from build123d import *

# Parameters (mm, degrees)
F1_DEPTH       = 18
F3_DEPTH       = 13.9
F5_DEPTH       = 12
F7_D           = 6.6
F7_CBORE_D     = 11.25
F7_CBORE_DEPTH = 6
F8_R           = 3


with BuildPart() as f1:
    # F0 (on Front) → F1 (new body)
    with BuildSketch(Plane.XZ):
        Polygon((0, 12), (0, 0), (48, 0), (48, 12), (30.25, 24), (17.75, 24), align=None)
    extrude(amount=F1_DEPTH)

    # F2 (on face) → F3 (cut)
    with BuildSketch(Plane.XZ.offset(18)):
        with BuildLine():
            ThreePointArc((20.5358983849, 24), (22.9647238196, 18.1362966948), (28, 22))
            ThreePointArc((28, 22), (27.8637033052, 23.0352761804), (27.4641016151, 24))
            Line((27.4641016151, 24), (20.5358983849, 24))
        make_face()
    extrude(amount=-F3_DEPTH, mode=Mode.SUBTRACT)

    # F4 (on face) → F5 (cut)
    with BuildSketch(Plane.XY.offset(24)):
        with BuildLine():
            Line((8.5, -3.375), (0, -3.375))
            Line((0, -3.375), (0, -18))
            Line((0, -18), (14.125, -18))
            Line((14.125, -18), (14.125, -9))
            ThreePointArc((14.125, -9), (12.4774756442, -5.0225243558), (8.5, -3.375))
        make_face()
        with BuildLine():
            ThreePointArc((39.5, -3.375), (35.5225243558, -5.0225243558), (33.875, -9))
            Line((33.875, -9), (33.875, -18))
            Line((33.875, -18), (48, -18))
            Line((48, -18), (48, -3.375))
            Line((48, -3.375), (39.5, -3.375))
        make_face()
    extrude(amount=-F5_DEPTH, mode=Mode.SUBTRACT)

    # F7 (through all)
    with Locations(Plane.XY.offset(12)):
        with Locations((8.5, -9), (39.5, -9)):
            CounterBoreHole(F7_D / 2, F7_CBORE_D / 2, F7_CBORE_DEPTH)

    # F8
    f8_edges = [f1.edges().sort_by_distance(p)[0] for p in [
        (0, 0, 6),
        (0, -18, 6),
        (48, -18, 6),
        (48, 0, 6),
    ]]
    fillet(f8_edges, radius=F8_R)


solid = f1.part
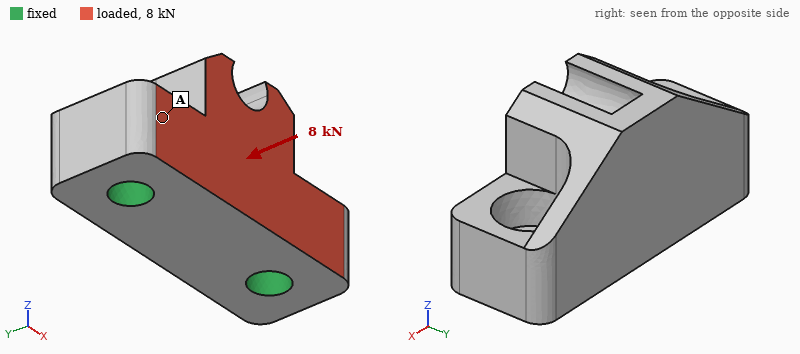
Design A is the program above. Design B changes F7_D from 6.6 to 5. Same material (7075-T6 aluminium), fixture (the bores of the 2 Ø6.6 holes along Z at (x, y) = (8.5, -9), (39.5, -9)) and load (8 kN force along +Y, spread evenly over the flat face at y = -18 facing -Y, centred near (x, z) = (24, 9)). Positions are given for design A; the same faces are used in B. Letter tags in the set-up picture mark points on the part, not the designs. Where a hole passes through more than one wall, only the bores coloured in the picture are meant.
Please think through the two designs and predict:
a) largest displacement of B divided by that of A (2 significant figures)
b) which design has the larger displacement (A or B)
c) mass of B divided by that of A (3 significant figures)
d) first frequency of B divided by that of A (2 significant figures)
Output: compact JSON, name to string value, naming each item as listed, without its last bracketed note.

{"largest displacement of B divided by that of A": "1.3", "which design has the larger displacement": "B", "mass of B divided by that of A": "1.01", "first frequency of B divided by that of A": "0.86"}
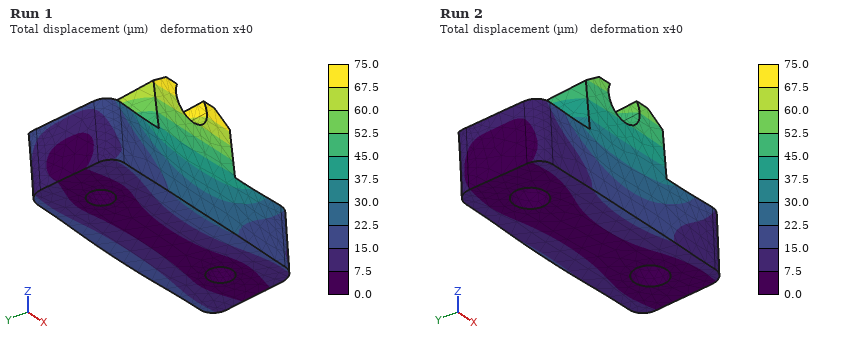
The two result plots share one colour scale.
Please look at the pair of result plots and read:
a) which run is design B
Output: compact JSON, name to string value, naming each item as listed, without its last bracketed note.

{"which run is design B": "Run 1"}
